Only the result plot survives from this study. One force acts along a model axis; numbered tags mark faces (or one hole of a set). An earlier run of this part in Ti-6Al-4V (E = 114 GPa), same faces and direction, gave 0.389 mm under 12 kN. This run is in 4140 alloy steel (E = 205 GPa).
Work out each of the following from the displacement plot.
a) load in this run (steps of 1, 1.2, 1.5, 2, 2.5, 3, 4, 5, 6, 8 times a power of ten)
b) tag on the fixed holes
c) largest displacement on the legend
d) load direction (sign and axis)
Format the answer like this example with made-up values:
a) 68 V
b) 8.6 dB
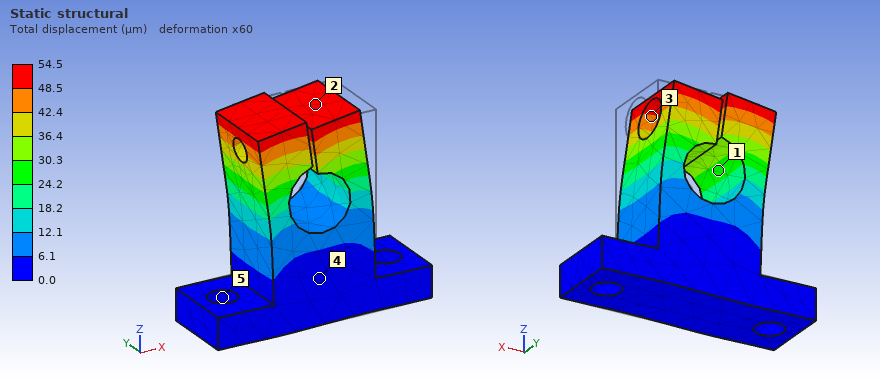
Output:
a) 3 kN
b) 5
c) 54.5 µm
d) -X
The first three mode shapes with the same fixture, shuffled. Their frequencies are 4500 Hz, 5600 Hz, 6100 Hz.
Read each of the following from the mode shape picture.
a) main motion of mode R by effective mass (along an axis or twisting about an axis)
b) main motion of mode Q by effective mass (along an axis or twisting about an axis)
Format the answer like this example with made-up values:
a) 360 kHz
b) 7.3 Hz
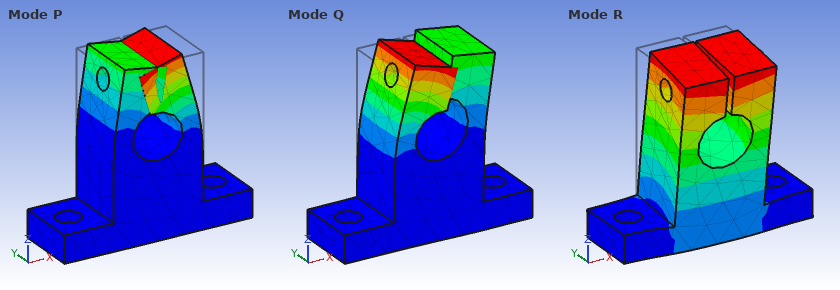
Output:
a) along Y
b) along X
